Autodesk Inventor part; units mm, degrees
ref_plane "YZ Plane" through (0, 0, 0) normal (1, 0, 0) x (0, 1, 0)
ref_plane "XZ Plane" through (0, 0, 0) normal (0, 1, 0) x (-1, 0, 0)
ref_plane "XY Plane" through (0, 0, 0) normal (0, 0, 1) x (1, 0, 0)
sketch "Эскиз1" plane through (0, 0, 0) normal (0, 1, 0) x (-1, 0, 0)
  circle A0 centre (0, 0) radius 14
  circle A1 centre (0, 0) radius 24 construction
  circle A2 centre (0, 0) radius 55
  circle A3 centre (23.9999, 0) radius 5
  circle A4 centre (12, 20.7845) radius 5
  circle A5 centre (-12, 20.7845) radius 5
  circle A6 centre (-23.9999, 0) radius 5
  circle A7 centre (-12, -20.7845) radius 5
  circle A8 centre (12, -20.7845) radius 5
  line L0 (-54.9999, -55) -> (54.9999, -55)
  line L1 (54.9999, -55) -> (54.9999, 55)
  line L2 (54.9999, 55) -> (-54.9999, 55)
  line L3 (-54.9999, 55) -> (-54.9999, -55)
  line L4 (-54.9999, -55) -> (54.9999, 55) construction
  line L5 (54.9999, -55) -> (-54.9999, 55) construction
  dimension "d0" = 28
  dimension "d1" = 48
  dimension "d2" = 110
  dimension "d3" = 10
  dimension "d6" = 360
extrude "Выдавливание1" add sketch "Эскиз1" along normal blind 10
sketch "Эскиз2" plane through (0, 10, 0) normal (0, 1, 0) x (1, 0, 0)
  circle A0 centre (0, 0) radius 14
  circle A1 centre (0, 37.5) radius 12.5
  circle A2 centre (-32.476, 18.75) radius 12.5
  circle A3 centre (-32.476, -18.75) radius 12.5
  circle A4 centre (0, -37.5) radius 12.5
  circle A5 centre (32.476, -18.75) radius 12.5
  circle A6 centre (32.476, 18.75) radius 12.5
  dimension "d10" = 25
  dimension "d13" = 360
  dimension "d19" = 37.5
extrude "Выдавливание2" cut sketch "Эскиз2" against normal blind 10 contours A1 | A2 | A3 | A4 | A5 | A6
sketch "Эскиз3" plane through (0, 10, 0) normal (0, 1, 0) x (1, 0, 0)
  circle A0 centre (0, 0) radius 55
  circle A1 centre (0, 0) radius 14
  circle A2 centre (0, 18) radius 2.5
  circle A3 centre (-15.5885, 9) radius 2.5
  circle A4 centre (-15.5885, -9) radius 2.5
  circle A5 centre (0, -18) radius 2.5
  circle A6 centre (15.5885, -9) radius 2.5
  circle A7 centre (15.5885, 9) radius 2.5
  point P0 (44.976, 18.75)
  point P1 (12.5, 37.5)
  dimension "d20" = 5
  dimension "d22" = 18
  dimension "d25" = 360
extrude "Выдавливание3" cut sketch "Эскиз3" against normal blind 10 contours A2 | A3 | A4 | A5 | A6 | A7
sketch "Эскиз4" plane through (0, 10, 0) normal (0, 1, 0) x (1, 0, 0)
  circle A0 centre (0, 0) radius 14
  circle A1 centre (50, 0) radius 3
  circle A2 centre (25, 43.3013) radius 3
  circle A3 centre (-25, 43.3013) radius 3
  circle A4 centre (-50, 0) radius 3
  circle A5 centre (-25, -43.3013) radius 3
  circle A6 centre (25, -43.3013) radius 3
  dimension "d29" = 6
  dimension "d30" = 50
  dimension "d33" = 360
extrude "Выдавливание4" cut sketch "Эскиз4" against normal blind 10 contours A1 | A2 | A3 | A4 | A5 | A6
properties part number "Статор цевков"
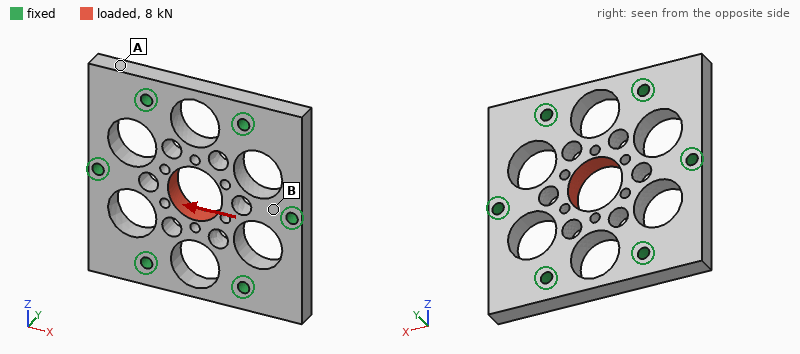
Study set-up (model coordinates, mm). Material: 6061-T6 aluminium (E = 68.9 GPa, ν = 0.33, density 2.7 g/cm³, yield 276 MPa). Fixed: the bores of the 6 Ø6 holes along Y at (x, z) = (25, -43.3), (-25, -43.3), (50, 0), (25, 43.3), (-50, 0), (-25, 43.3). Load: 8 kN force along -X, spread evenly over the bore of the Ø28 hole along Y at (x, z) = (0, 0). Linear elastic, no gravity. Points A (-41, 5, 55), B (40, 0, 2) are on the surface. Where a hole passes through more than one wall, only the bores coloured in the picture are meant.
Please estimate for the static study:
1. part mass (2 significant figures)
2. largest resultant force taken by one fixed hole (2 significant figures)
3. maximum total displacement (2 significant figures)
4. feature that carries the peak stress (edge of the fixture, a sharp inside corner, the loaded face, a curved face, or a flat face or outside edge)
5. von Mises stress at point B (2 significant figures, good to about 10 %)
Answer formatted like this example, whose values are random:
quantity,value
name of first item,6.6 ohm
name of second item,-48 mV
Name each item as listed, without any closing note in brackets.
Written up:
quantity,value
part mass,210 g
largest resultant force taken by one fixed hole,2.3 kN
maximum total displacement,14 µm
feature that carries the peak stress,a curved face
von Mises stress at point B,18 MPa
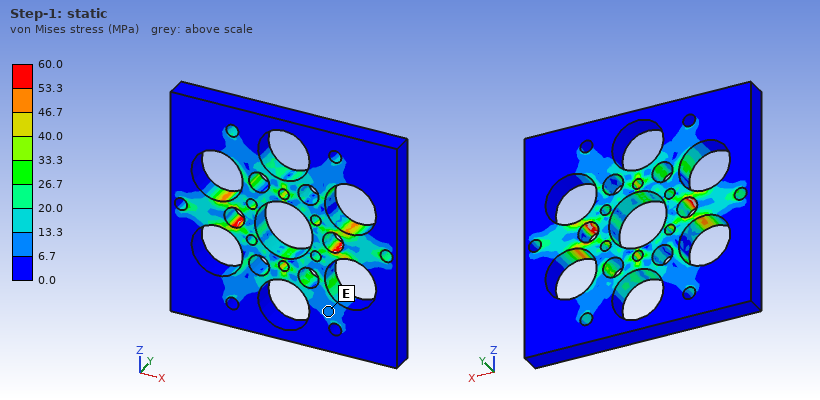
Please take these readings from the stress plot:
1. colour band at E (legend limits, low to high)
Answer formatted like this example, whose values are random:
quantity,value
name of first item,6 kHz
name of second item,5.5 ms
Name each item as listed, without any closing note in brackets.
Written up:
quantity,value
colour band at E,6.7 to 13.3 MPa
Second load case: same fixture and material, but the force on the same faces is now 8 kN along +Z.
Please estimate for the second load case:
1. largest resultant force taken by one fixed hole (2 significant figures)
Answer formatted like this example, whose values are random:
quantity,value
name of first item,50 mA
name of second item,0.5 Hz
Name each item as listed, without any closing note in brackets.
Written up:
quantity,value
largest resultant force taken by one fixed hole,2.0 kN
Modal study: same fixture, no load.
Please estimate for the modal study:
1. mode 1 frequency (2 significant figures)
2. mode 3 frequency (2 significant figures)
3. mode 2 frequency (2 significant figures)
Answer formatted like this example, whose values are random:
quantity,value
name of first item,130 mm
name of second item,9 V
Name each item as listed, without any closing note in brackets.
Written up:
quantity,value
mode 1 frequency,7700 Hz
mode 3 frequency,9400 Hz
mode 2 frequency,9300 Hz
